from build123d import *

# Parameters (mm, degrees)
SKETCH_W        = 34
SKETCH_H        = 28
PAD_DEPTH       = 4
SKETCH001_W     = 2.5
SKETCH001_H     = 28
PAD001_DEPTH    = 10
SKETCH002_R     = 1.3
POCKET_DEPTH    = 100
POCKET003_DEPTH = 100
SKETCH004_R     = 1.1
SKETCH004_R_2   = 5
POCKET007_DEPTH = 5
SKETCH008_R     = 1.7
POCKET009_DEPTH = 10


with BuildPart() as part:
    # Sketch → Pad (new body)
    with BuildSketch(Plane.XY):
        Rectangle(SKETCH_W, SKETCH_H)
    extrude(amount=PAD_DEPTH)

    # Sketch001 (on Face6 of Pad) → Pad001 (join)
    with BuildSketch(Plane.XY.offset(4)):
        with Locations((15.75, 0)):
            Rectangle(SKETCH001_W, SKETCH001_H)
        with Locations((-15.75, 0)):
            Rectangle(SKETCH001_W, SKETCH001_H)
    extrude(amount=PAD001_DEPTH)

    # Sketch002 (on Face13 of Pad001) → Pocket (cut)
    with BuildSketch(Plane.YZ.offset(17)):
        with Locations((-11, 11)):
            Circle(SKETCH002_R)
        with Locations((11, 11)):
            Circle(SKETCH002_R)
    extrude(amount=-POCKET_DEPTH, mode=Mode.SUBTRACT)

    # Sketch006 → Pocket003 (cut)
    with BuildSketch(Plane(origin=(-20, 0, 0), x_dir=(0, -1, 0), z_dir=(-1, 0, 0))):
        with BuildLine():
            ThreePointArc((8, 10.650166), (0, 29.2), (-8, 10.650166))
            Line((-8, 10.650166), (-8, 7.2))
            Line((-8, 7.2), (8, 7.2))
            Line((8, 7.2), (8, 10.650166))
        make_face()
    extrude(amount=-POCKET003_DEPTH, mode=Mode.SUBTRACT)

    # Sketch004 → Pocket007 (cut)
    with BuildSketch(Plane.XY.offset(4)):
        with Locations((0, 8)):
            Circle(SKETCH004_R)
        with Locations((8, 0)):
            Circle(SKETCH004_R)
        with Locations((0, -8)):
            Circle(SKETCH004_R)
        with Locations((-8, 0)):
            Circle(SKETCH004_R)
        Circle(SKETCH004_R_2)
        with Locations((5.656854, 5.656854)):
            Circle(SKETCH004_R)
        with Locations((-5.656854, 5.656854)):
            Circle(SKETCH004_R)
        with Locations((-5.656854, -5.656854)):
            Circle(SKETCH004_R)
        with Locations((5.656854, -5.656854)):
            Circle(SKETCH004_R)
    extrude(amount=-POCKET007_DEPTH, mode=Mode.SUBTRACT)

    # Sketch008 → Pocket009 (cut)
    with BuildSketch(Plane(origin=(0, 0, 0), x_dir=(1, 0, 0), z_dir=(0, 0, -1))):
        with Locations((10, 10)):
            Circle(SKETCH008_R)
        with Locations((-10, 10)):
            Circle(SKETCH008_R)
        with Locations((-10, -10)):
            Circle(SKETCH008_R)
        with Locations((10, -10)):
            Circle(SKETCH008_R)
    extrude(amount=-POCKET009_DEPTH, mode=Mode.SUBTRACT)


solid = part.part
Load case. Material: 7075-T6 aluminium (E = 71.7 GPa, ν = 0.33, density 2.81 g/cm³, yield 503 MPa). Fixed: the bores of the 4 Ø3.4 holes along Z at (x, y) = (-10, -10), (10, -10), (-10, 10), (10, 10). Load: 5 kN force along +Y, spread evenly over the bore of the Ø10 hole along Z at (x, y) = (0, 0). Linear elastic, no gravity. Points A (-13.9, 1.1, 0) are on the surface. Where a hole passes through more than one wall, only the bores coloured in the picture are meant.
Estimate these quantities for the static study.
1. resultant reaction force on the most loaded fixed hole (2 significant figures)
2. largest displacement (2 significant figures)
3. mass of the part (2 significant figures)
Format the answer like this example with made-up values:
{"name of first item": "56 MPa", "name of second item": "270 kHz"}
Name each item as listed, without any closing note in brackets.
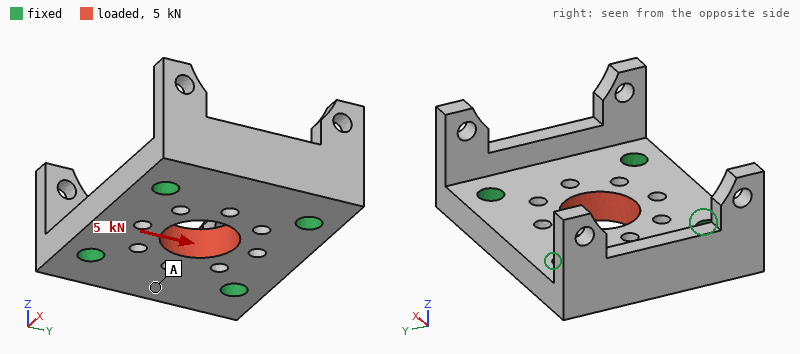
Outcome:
{"resultant reaction force on the most loaded fixed hole": "1.3 kN", "largest displacement": "10 µm", "mass of the part": "11 g"}
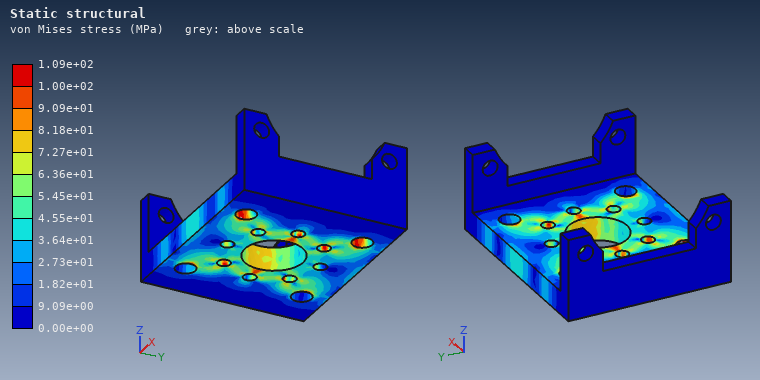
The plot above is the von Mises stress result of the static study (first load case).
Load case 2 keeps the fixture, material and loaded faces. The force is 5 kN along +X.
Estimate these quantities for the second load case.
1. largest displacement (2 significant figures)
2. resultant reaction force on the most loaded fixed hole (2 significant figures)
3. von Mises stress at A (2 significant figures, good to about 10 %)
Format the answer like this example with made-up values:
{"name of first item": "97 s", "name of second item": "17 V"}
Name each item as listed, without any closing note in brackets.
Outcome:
{"largest displacement": "8.9 µm", "resultant reaction force on the most loaded fixed hole": "1.3 kN", "von Mises stress at A": "17 MPa"}
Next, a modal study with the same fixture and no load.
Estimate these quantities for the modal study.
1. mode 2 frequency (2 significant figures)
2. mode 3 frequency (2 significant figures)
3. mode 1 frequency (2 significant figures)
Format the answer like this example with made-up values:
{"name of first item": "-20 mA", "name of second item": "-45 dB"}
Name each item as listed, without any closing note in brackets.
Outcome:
{"mode 2 frequency": "18 kHz", "mode 3 frequency": "19 kHz", "mode 1 frequency": "18 kHz"}
